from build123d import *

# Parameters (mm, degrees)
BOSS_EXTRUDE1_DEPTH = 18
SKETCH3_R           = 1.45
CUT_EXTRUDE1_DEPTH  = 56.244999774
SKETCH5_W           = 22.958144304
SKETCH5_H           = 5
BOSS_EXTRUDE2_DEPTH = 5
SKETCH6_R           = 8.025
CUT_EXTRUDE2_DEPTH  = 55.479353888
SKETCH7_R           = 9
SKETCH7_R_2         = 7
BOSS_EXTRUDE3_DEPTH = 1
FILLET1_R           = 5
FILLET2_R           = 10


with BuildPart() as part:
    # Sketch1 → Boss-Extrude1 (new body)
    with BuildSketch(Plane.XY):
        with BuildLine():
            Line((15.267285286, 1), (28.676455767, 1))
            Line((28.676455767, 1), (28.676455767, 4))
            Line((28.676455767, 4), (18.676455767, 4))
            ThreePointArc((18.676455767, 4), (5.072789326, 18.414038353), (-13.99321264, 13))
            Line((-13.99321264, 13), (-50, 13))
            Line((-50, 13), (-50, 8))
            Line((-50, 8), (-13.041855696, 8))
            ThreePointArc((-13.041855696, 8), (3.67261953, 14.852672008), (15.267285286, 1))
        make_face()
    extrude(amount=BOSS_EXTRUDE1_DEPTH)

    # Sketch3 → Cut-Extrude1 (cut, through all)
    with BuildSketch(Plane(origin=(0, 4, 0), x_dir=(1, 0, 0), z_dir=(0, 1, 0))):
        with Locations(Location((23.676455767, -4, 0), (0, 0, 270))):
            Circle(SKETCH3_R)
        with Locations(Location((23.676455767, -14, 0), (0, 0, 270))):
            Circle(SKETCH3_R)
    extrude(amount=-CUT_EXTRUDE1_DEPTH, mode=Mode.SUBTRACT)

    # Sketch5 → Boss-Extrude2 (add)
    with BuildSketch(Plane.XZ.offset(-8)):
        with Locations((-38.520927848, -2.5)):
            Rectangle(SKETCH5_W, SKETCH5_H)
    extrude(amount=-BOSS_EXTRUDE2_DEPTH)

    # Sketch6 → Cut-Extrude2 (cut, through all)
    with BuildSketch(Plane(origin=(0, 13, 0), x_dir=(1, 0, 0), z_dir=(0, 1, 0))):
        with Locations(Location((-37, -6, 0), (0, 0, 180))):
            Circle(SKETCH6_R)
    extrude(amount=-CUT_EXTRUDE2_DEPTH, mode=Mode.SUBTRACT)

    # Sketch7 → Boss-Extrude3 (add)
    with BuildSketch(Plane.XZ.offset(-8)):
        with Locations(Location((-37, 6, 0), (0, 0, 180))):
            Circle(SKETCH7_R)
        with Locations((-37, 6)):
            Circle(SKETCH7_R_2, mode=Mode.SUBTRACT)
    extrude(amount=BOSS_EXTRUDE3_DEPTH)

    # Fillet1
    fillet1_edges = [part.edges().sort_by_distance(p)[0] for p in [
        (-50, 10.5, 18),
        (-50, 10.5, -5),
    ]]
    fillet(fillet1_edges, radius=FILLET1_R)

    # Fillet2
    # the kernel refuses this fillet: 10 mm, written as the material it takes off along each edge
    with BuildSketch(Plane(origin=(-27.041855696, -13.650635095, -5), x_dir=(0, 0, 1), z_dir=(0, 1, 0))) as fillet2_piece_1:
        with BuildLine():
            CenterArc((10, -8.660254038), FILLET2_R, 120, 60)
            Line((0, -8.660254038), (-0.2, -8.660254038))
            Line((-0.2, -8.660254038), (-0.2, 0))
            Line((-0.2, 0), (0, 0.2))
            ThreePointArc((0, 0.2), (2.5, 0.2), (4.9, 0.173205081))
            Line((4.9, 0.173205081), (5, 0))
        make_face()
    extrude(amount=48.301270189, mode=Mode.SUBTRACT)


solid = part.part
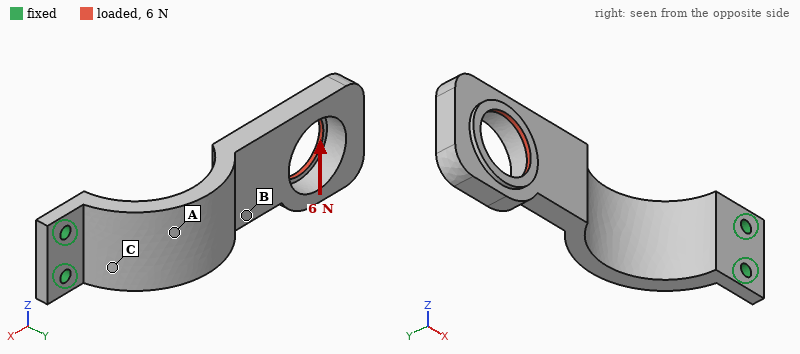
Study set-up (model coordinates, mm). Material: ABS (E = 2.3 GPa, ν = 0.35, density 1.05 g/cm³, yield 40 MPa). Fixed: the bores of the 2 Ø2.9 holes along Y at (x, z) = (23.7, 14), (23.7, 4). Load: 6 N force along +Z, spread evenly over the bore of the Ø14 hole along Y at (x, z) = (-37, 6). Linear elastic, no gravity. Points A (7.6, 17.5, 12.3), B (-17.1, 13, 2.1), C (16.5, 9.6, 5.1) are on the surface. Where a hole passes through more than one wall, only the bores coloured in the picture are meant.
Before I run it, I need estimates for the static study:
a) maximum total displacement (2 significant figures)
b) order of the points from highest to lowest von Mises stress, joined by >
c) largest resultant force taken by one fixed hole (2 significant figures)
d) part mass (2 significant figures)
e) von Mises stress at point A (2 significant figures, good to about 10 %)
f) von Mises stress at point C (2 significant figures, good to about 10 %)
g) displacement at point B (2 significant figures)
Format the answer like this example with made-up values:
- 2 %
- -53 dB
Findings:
- 0.97 mm
- C > A > B
- 32 N
- 6.5 g
- 3.0 MPa
- 4.7 MPa
- 0.42 mm
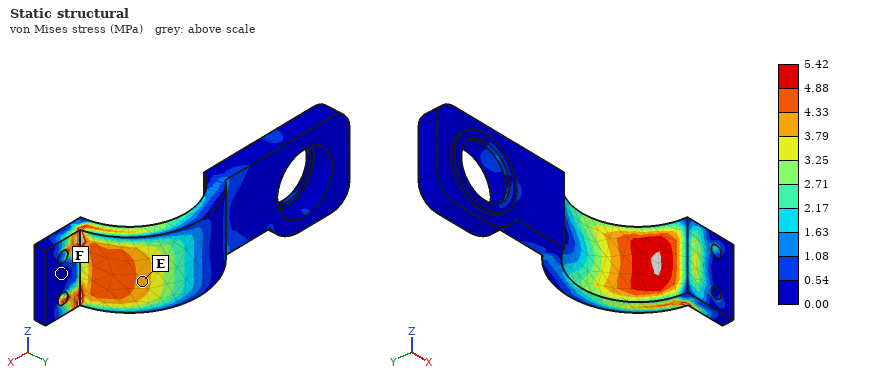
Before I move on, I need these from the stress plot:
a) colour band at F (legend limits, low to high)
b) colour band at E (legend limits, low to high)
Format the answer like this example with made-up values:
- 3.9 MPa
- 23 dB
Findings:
- 0.00 to 0.54 MPa
- 3.79 to 4.33 MPa
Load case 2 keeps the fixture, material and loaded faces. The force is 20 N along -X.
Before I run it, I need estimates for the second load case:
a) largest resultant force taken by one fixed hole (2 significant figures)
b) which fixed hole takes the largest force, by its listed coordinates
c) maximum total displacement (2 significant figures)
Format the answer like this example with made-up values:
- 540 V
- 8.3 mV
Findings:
- 15 N
- (23.7, 4)
- 0.90 mm
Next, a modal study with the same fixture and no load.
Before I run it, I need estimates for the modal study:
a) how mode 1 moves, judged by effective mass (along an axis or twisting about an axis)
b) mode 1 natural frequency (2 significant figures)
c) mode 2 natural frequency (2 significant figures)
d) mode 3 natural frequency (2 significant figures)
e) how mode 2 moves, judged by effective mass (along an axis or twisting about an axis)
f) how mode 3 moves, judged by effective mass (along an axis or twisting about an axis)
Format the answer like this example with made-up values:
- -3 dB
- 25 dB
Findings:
- along Y
- 130 Hz
- 280 Hz
- 670 Hz
- along Z
- along X
